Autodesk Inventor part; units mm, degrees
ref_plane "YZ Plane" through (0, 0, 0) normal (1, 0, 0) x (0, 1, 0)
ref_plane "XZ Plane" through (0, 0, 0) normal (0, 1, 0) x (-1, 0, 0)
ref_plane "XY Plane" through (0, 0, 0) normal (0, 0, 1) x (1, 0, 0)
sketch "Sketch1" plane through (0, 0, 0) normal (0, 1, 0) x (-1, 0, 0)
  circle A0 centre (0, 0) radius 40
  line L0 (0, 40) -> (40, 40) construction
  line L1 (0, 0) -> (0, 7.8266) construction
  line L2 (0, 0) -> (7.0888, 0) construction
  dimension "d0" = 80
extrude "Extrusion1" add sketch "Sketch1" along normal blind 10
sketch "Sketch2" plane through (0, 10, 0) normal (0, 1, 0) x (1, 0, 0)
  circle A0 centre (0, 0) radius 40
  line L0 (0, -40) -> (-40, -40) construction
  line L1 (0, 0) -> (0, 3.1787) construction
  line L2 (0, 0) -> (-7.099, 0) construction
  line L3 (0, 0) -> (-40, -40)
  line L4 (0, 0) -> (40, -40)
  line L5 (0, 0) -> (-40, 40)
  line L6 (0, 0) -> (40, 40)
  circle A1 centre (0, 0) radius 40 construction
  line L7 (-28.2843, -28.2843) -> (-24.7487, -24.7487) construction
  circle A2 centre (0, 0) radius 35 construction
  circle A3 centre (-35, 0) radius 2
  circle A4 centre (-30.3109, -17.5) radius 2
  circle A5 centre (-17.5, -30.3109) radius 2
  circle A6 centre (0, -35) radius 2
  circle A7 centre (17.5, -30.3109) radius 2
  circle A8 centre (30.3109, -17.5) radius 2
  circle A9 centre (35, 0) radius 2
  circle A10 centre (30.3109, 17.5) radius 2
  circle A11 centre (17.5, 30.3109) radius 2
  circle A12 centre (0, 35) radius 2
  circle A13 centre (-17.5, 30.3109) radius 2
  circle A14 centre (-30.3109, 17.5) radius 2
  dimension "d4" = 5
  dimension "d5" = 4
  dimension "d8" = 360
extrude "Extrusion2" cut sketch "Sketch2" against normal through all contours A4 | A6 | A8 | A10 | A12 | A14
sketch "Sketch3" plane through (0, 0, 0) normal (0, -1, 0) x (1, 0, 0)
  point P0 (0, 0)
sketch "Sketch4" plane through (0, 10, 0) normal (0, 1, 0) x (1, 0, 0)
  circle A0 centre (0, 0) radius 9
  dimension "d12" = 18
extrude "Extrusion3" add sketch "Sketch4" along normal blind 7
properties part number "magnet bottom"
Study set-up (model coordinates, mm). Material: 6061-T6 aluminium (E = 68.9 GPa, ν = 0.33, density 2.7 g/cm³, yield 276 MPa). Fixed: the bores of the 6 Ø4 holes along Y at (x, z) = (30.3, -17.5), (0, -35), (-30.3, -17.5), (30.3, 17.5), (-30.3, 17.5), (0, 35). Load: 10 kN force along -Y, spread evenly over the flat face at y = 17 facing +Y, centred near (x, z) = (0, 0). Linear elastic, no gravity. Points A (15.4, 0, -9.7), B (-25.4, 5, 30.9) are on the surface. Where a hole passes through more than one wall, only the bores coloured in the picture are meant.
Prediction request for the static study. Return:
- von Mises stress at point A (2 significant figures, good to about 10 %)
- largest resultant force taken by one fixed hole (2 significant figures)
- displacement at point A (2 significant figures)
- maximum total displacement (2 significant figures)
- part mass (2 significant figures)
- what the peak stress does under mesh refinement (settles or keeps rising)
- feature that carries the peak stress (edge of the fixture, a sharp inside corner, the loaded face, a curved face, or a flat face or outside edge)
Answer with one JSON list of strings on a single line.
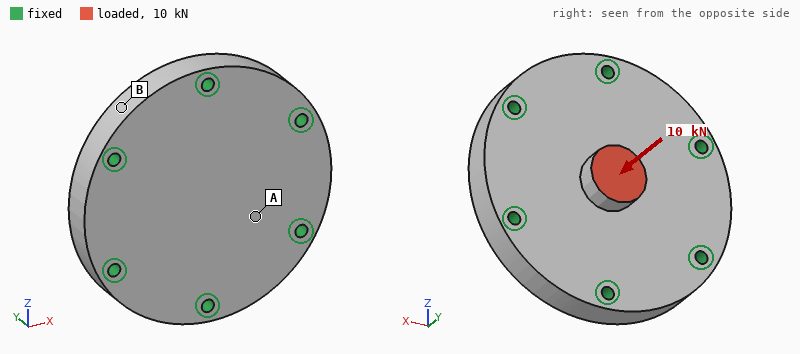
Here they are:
["29 MPa", "1.7 kN", "27 µm", "49 µm", "140 g", "keeps rising", "edge of the fixture"]
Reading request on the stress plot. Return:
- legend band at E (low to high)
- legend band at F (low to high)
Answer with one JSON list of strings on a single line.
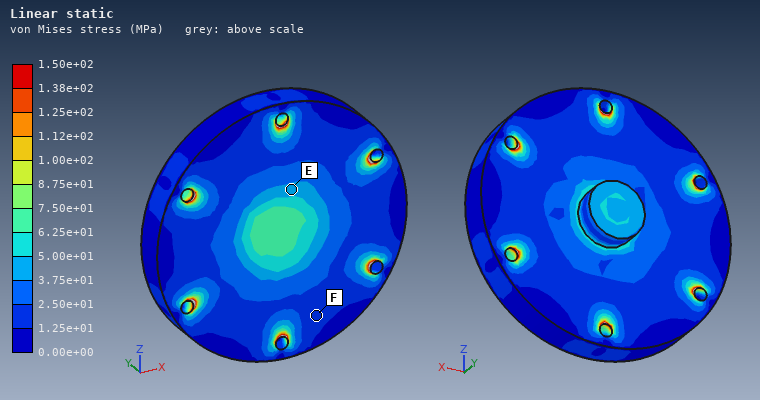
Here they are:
["3.75e+01 to 5.00e+01 MPa", "1.25e+01 to 2.50e+01 MPa"]
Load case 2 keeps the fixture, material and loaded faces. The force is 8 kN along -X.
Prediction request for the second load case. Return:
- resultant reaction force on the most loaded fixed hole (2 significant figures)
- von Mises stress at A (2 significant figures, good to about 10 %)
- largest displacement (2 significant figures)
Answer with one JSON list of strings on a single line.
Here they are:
["2.0 kN", "17 MPa", "42 µm"]
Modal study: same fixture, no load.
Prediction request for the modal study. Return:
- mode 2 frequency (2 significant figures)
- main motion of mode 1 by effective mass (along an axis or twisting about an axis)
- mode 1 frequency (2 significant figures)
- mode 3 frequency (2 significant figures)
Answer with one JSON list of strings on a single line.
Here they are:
["23 kHz", "along Y", "13 kHz", "23 kHz"]
